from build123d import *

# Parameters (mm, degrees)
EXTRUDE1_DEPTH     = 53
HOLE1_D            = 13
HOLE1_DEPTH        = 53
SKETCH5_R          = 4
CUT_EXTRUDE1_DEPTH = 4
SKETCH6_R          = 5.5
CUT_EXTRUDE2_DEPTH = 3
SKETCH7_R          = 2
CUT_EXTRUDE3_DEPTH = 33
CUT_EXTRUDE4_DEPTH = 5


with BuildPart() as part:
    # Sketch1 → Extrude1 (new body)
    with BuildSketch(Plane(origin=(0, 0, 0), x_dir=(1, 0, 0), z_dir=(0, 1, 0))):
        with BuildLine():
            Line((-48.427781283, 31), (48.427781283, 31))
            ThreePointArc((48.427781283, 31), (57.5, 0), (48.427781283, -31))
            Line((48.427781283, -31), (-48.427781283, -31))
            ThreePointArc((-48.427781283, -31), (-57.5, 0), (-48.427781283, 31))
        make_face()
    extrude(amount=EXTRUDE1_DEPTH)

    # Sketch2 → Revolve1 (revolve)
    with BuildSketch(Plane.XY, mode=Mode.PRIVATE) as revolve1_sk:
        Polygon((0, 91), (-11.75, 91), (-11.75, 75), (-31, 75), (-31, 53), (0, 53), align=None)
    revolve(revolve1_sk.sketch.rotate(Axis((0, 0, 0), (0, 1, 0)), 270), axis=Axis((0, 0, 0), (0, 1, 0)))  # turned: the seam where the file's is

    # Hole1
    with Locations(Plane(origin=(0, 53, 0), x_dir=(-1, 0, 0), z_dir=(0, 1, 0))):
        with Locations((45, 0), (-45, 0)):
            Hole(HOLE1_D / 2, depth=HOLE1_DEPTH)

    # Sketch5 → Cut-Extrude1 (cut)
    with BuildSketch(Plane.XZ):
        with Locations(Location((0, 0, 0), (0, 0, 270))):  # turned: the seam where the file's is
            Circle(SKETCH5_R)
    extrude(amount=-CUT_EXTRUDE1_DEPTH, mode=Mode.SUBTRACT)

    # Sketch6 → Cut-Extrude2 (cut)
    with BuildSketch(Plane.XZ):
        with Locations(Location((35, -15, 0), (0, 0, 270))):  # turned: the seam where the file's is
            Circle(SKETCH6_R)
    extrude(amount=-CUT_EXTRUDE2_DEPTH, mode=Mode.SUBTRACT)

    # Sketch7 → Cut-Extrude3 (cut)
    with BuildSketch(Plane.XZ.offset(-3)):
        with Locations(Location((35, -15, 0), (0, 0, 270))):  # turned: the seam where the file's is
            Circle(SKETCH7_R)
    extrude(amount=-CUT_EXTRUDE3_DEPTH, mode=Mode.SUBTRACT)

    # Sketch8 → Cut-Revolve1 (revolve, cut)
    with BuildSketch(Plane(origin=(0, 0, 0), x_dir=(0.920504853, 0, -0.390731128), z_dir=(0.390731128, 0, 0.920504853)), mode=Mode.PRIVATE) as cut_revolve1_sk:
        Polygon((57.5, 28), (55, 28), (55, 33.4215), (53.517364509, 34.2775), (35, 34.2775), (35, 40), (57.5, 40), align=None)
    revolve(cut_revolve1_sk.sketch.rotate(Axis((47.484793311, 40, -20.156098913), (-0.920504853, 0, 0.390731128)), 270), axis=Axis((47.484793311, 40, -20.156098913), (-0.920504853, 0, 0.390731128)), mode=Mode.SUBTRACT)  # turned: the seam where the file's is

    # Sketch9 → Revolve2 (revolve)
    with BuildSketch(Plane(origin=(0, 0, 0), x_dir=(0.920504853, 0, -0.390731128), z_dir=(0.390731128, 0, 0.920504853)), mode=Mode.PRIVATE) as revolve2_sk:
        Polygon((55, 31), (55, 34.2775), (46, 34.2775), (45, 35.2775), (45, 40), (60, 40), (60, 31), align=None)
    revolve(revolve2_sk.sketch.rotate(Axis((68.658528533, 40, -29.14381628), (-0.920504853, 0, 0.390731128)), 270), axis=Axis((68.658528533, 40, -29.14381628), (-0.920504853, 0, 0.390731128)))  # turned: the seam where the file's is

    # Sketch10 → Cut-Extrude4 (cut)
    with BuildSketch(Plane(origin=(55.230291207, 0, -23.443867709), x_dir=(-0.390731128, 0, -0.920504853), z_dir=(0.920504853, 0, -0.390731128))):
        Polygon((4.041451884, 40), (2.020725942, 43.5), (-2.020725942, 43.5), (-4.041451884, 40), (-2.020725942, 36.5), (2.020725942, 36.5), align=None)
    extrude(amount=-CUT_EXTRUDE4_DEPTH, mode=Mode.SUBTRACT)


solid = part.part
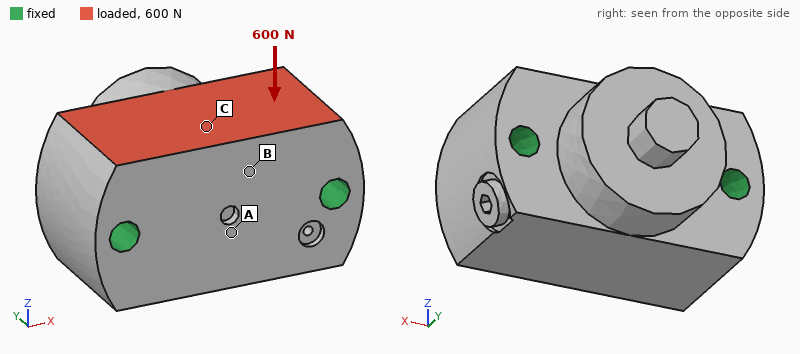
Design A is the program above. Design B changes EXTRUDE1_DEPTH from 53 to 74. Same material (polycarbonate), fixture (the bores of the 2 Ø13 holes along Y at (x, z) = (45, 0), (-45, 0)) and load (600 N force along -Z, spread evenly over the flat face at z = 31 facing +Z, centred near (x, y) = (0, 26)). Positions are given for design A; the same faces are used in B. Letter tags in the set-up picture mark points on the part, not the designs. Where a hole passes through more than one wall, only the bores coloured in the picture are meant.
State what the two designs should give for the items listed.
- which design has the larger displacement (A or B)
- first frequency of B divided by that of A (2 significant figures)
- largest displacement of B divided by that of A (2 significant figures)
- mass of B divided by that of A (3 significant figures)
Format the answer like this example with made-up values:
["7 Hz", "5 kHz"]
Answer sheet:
["A", "1.5", "0.76", "1.18"]
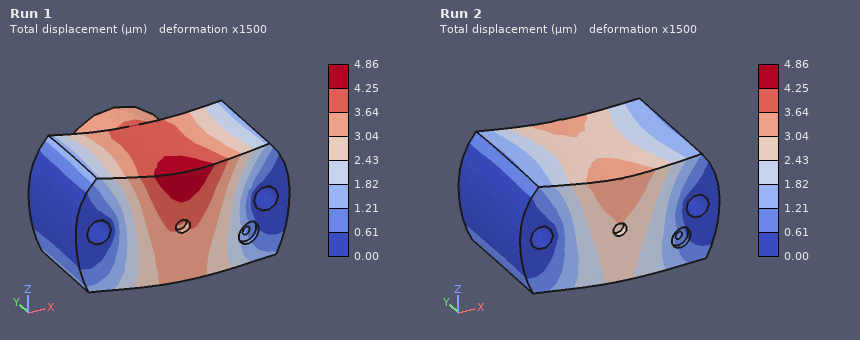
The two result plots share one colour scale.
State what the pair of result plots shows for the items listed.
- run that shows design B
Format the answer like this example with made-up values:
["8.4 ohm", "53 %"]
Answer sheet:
["Run 2"]
